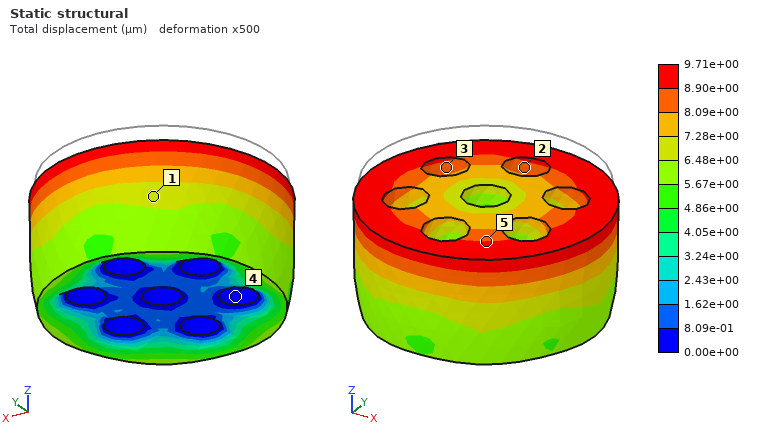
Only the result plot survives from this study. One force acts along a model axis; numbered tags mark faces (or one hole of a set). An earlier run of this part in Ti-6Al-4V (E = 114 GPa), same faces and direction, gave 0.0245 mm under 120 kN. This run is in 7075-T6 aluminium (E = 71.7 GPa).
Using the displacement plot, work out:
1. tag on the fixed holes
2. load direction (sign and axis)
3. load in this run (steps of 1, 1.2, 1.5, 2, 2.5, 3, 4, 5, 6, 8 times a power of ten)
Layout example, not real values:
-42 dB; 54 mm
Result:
4; -Z; 30 kN
